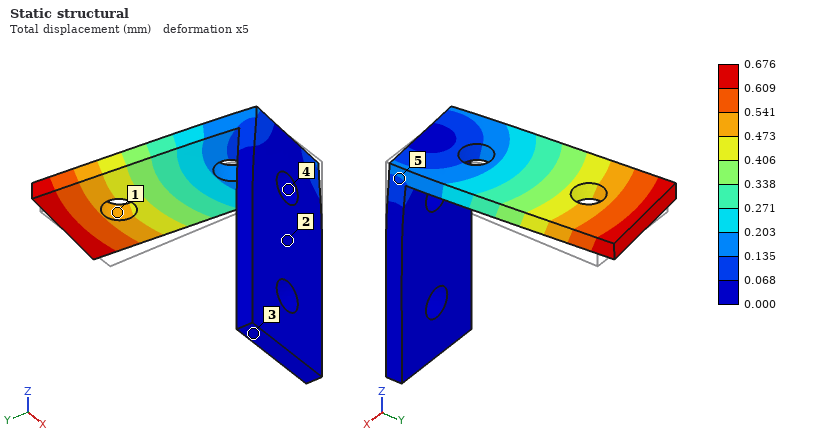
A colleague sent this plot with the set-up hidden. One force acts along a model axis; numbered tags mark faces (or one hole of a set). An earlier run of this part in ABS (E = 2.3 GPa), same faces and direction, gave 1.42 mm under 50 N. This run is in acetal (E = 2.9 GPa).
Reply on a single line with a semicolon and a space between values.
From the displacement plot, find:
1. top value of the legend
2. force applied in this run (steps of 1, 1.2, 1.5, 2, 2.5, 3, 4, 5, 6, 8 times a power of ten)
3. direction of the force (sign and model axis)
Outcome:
0.676 mm; 30 N; -X
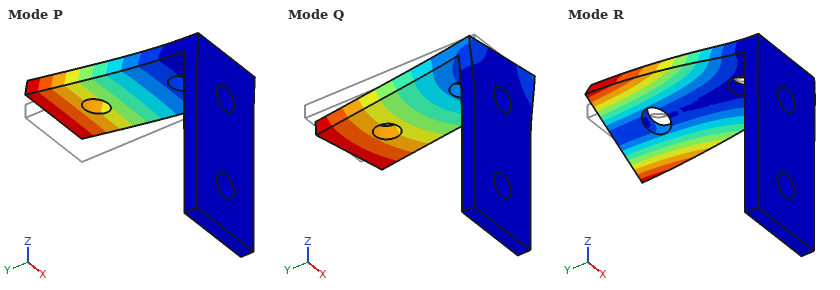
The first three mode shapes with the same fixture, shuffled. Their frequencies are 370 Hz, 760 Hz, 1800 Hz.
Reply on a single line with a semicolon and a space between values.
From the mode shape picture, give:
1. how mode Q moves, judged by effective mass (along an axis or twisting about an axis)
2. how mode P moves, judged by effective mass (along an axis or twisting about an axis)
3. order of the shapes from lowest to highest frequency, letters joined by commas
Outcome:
along X; along Z; P, Q, R
